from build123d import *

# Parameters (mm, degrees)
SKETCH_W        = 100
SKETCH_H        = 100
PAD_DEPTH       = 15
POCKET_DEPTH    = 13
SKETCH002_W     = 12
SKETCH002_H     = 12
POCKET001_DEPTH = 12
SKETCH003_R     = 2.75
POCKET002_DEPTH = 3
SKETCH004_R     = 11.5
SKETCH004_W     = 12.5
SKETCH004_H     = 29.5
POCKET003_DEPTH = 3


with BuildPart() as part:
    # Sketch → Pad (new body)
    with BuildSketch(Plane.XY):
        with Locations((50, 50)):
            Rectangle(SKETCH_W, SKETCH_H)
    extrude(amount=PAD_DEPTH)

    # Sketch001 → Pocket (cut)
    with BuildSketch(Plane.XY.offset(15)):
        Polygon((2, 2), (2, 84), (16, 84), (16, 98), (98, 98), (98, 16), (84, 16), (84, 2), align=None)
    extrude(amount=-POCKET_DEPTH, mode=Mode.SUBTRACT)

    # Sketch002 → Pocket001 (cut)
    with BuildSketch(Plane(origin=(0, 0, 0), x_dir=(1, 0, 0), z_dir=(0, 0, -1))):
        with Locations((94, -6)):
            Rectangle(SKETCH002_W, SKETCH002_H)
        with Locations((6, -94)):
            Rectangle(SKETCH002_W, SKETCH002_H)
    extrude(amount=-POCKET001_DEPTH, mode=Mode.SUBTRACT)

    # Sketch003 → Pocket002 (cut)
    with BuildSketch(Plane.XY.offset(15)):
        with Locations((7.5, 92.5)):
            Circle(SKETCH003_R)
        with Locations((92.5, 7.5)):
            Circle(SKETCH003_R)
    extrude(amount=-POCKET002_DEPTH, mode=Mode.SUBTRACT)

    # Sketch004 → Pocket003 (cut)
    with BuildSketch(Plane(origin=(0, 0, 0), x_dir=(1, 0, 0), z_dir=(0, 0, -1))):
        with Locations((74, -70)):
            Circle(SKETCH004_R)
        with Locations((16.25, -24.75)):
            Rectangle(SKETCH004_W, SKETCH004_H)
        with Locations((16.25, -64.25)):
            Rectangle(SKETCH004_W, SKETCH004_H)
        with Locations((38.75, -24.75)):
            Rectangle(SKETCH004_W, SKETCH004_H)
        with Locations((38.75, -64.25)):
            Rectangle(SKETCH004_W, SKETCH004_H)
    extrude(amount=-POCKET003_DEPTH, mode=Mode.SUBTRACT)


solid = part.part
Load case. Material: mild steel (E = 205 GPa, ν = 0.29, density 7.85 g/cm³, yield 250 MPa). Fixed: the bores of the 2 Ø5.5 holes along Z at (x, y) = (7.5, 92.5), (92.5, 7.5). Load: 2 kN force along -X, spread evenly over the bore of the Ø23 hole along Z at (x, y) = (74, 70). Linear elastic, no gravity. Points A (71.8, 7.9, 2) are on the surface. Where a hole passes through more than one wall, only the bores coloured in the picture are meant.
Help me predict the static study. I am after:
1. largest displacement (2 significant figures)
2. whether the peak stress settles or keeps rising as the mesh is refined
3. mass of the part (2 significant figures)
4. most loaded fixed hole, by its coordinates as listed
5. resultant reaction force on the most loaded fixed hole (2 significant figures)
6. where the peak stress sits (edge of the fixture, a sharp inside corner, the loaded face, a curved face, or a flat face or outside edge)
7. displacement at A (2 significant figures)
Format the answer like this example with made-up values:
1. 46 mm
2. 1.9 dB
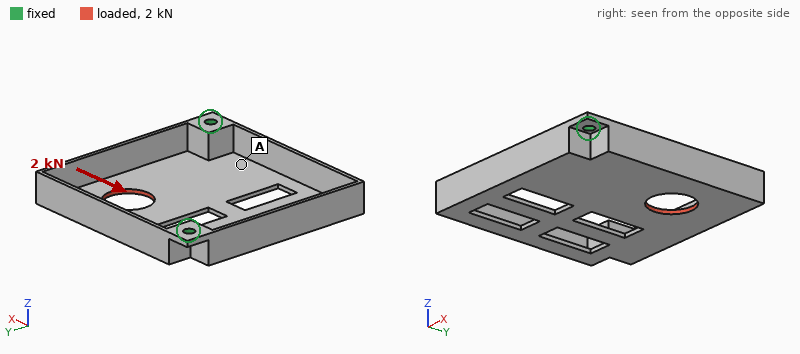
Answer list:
1. 0.13 mm
2. keeps rising
3. 220 g
4. (7.5, 92.5)
5. 1.3 kN
6. edge of the fixture
7. 0.028 mm
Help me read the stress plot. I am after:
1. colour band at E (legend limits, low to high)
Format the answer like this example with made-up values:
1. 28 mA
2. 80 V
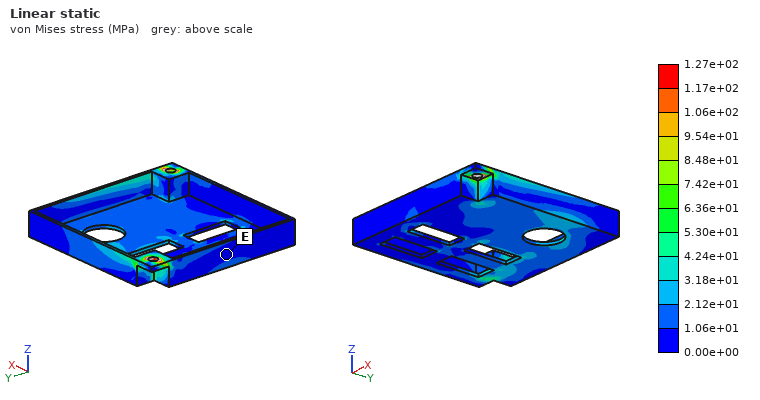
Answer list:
1. 0.00e+00 to 1.06e+01 MPa
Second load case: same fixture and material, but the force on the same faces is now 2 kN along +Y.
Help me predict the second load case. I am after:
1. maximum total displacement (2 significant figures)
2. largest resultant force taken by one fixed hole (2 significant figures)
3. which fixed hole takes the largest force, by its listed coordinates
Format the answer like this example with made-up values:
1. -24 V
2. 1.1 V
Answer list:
1. 0.14 mm
2. 1.4 kN
3. (92.5, 7.5)
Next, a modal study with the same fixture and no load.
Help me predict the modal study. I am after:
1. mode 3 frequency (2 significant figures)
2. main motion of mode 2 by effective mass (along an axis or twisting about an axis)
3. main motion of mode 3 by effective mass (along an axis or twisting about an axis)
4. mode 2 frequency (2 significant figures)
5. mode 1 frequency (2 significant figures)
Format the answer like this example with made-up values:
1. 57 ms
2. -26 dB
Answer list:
1. 1800 Hz
2. along Z
3. along Z
4. 1200 Hz
5. 930 Hz
